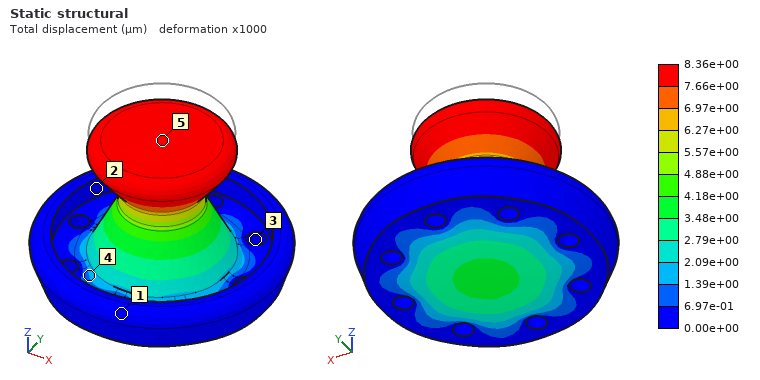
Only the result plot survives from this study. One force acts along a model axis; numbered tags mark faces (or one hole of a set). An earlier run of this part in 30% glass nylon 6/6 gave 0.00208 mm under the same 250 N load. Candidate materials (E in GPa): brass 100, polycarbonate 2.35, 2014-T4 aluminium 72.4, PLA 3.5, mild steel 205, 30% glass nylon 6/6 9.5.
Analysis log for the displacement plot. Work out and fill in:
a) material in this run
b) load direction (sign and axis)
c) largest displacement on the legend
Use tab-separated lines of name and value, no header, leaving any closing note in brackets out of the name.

material in this run	polycarbonate
load direction	-Z
largest displacement on the legend	8.36e+00 µm
